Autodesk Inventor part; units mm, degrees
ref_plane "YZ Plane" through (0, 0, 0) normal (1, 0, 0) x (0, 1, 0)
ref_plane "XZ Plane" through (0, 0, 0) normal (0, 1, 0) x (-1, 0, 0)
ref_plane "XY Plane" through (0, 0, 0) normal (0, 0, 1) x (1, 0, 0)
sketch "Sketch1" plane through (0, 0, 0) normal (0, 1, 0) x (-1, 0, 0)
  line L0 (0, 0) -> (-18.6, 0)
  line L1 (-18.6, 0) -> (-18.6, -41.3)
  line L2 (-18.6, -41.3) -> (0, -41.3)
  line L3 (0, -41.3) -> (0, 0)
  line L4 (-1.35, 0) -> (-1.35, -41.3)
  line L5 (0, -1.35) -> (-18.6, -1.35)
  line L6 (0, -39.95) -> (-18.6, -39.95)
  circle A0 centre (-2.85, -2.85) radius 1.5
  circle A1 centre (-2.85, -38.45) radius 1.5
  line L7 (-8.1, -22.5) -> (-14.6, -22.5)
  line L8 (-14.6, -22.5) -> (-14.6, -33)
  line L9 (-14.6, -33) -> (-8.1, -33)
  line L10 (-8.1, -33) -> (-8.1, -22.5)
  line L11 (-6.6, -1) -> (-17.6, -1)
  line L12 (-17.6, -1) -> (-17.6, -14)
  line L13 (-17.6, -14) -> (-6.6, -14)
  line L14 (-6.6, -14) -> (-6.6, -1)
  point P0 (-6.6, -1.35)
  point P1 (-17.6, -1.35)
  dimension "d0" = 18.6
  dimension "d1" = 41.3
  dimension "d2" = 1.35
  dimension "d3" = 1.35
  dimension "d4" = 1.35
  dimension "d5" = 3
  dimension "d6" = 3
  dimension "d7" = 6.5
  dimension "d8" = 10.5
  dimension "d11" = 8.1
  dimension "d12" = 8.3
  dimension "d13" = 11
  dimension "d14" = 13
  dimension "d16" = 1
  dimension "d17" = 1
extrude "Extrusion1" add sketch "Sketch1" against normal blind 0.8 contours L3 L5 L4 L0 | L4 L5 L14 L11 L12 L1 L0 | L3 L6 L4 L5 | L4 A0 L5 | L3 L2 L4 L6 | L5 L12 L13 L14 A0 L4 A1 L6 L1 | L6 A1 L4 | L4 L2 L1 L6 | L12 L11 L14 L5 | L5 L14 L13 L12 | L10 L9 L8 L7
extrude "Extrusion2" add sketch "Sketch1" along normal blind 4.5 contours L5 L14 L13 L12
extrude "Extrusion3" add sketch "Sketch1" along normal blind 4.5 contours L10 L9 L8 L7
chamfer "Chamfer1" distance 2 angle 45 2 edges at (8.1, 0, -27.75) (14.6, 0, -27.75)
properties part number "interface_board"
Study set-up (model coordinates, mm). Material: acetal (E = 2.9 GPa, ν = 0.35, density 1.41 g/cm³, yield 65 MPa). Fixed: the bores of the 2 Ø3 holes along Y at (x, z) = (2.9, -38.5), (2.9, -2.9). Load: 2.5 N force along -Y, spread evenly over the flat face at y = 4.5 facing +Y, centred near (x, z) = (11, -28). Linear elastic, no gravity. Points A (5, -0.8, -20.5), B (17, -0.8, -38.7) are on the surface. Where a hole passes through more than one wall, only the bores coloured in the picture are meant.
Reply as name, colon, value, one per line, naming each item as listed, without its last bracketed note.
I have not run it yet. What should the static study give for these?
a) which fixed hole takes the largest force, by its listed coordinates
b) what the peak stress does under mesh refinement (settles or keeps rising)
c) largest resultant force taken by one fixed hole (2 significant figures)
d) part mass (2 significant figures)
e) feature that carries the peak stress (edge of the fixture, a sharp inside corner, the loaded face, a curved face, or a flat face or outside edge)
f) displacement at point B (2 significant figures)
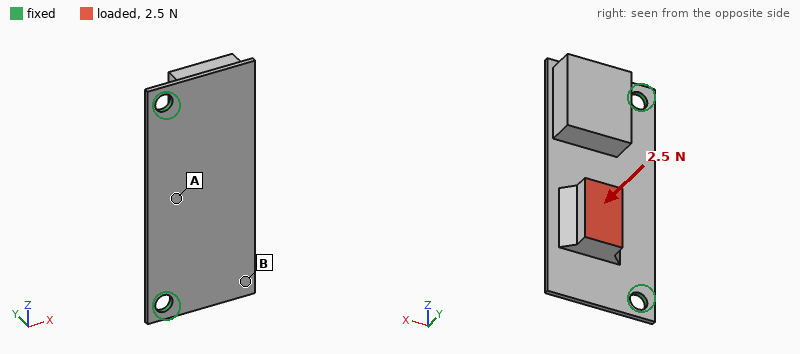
which fixed hole takes the largest force, by its listed coordinates: (2.9, -38.5)
what the peak stress does under mesh refinement: keeps rising
largest resultant force taken by one fixed hole: 1.7 N
part mass: 2.2 g
feature that carries the peak stress: edge of the fixture
displacement at point B: 0.28 mm
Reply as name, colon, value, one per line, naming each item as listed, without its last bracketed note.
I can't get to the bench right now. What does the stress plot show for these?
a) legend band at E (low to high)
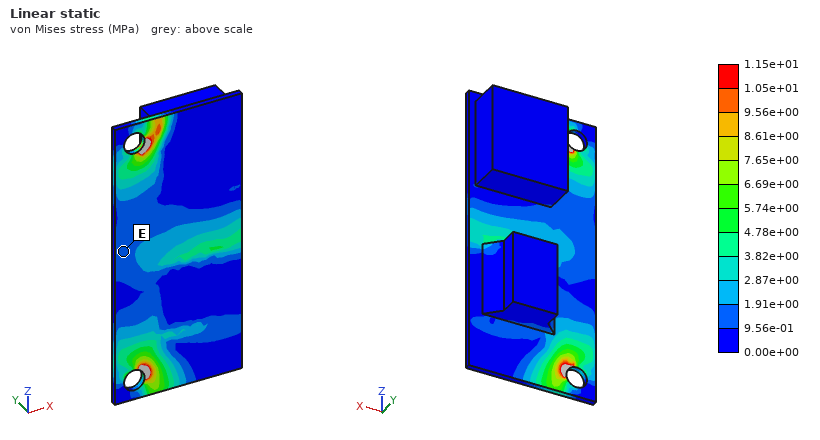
legend band at E: 9.56e-01 to 1.91e+00 MPa
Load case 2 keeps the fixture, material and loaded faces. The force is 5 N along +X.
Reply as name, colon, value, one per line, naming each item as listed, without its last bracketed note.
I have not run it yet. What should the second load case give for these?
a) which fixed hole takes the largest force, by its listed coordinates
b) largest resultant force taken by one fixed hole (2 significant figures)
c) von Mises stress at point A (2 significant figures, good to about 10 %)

which fixed hole takes the largest force, by its listed coordinates: (2.9, -38.5)
largest resultant force taken by one fixed hole: 3.8 N
von Mises stress at point A: 1.4 MPa
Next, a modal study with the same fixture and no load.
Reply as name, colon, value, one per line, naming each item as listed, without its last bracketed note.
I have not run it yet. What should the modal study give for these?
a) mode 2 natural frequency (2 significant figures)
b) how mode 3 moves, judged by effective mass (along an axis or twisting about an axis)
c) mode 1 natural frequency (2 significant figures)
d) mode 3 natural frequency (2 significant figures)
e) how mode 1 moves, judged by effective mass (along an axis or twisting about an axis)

mode 2 natural frequency: 960 Hz
how mode 3 moves, judged by effective mass: twisting about X
mode 1 natural frequency: 350 Hz
mode 3 natural frequency: 1100 Hz
how mode 1 moves, judged by effective mass: along Y
